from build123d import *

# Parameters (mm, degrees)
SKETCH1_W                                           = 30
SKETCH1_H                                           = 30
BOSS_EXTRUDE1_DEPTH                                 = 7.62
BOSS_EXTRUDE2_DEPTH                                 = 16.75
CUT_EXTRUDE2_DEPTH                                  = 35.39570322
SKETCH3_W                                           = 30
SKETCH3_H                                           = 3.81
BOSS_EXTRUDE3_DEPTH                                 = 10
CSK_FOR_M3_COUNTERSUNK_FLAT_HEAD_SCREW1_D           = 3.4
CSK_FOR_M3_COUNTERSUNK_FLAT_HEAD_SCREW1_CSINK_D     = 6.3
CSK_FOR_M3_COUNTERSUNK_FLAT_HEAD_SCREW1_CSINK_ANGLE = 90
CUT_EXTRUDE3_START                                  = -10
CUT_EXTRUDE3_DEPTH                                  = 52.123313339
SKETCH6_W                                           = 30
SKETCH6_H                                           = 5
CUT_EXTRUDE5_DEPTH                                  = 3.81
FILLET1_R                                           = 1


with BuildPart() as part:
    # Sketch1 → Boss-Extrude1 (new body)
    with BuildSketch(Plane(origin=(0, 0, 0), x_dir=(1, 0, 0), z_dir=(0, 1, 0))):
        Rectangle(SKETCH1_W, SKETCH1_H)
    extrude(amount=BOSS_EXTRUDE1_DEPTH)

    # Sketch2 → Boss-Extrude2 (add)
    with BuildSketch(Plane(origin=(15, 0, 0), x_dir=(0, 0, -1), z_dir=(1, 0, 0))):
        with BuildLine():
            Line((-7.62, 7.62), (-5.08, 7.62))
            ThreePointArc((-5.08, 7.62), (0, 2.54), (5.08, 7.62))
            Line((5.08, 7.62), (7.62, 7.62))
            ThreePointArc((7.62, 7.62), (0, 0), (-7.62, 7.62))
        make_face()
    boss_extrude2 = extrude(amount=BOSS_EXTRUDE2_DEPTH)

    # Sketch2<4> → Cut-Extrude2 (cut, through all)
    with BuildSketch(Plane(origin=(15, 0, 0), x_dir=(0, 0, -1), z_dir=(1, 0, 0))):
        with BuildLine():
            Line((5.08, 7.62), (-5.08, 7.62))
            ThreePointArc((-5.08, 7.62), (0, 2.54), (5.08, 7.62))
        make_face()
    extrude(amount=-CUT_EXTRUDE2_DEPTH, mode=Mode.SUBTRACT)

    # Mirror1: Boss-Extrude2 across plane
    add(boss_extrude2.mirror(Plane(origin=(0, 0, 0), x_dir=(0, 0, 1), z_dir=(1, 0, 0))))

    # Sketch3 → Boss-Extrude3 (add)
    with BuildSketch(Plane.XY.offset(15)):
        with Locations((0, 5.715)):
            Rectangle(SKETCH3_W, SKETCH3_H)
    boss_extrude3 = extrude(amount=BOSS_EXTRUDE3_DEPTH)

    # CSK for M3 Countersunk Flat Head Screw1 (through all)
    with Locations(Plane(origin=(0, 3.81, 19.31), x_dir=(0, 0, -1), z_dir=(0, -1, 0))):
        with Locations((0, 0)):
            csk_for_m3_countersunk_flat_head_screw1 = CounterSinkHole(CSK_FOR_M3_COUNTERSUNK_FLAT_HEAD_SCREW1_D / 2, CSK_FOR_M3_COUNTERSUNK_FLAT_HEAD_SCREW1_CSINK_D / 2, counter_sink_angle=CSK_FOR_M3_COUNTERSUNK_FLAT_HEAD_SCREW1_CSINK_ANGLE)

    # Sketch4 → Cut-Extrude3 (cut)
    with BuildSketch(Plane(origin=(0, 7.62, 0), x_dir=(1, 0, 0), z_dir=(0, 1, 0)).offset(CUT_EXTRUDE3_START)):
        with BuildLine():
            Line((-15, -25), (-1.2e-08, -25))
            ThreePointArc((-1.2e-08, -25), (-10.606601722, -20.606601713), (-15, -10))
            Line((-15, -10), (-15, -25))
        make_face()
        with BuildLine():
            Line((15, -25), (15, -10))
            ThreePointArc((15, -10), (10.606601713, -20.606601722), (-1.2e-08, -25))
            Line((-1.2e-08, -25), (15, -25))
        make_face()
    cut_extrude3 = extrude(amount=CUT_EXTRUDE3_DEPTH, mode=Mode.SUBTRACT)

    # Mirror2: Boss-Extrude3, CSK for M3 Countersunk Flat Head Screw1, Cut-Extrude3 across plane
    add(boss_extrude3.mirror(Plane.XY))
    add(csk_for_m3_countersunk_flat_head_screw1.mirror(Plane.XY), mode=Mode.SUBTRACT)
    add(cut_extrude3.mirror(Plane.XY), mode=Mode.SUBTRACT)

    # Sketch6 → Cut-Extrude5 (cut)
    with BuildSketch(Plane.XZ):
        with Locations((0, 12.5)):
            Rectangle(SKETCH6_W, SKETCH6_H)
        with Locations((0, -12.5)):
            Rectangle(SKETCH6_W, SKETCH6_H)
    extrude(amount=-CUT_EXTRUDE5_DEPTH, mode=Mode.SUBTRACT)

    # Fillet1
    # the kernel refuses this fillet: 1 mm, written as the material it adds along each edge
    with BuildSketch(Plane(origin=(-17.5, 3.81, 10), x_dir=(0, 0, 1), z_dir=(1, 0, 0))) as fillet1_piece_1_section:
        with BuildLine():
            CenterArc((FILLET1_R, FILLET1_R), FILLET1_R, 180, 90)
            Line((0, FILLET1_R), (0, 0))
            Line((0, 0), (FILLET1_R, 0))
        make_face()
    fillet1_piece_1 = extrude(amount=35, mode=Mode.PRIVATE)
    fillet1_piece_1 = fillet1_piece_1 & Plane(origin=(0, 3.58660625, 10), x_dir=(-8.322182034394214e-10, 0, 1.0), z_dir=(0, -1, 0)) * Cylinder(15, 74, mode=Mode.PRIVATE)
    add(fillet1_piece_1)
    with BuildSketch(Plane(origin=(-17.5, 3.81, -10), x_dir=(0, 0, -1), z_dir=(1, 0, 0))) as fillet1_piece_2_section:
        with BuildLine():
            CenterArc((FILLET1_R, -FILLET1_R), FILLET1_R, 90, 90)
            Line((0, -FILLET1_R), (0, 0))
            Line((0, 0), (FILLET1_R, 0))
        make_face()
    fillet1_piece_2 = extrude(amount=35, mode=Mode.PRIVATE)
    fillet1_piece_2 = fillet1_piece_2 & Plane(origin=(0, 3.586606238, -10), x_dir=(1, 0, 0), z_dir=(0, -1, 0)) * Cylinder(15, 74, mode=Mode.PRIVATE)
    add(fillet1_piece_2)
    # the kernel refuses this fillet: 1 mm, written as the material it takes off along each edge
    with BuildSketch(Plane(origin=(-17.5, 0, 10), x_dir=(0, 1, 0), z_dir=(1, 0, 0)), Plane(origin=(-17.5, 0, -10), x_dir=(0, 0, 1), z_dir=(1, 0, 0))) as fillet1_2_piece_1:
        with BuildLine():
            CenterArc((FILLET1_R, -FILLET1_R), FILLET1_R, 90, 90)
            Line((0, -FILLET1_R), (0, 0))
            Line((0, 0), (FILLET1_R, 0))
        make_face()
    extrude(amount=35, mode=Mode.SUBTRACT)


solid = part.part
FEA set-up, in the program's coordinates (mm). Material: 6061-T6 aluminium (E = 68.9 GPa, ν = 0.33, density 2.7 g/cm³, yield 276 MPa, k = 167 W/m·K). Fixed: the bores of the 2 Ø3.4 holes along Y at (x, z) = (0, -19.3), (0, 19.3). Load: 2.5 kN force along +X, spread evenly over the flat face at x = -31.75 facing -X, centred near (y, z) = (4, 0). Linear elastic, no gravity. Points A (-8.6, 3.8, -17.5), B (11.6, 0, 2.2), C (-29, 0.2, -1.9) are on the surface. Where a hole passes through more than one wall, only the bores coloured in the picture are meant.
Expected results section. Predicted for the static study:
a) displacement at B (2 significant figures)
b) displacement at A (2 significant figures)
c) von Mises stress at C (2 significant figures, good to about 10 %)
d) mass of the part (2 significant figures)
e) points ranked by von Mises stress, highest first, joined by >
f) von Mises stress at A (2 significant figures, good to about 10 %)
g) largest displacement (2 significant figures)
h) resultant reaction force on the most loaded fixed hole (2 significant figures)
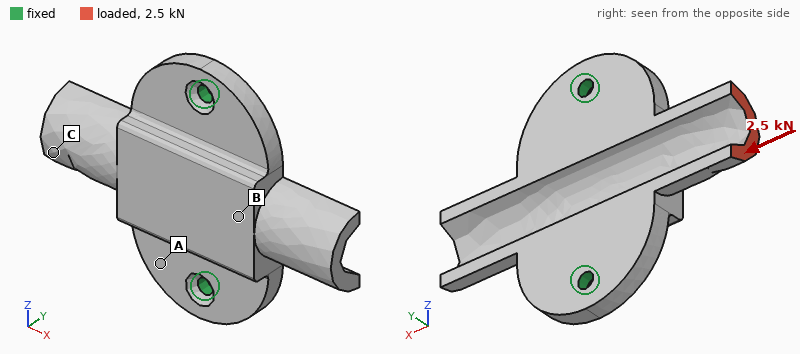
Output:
0.073 mm
0.027 mm
57 MPa
21 g
C > A > B
34 MPa
0.17 mm
1.3 kN
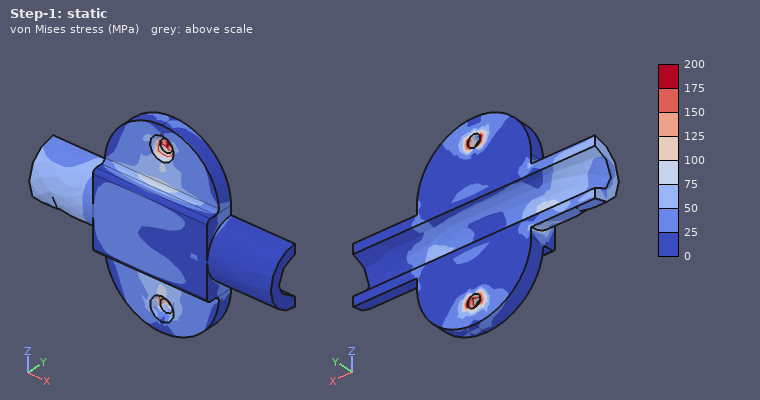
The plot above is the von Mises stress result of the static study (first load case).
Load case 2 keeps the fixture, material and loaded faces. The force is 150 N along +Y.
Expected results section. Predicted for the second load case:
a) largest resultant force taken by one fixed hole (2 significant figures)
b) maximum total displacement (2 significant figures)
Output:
190 N
0.15 mm
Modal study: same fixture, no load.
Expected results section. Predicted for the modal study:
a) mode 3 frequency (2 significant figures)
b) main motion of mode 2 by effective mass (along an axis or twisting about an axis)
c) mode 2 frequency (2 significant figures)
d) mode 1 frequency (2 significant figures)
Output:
11 kHz
along Y
6800 Hz
3100 Hz
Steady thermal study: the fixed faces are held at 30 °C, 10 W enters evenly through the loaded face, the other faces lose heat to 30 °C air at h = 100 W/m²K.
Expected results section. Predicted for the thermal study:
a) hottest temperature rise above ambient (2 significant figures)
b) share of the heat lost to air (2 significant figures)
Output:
27 K
25 %
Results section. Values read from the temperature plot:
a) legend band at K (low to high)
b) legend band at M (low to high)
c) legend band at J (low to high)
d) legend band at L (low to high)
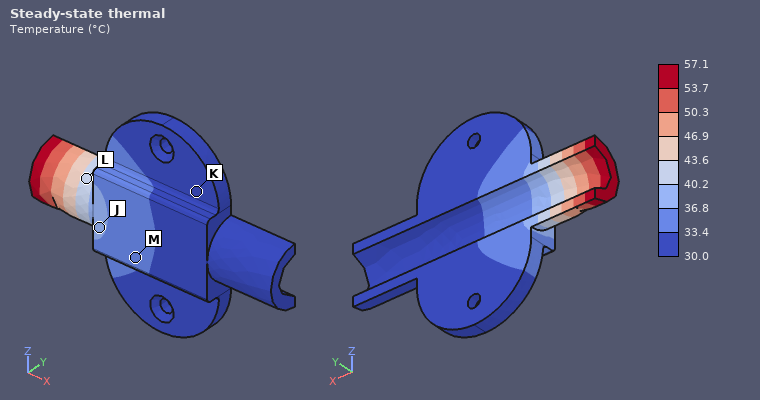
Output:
30.0 to 33.4 °C
33.4 to 36.8 °C
36.8 to 40.2 °C
40.2 to 43.6 °C
